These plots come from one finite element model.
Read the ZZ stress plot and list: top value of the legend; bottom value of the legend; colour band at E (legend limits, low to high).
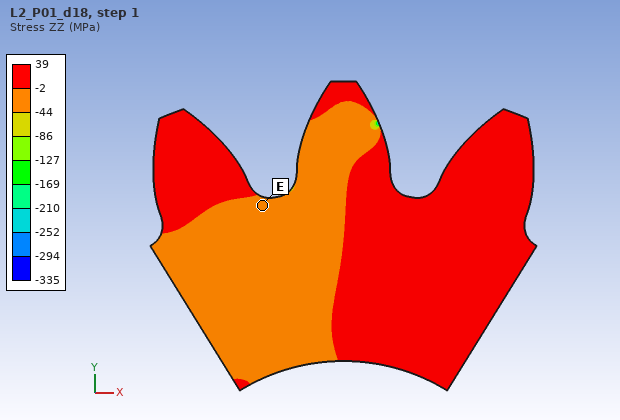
39 MPa
-335 MPa
-44 to -2 MPa
